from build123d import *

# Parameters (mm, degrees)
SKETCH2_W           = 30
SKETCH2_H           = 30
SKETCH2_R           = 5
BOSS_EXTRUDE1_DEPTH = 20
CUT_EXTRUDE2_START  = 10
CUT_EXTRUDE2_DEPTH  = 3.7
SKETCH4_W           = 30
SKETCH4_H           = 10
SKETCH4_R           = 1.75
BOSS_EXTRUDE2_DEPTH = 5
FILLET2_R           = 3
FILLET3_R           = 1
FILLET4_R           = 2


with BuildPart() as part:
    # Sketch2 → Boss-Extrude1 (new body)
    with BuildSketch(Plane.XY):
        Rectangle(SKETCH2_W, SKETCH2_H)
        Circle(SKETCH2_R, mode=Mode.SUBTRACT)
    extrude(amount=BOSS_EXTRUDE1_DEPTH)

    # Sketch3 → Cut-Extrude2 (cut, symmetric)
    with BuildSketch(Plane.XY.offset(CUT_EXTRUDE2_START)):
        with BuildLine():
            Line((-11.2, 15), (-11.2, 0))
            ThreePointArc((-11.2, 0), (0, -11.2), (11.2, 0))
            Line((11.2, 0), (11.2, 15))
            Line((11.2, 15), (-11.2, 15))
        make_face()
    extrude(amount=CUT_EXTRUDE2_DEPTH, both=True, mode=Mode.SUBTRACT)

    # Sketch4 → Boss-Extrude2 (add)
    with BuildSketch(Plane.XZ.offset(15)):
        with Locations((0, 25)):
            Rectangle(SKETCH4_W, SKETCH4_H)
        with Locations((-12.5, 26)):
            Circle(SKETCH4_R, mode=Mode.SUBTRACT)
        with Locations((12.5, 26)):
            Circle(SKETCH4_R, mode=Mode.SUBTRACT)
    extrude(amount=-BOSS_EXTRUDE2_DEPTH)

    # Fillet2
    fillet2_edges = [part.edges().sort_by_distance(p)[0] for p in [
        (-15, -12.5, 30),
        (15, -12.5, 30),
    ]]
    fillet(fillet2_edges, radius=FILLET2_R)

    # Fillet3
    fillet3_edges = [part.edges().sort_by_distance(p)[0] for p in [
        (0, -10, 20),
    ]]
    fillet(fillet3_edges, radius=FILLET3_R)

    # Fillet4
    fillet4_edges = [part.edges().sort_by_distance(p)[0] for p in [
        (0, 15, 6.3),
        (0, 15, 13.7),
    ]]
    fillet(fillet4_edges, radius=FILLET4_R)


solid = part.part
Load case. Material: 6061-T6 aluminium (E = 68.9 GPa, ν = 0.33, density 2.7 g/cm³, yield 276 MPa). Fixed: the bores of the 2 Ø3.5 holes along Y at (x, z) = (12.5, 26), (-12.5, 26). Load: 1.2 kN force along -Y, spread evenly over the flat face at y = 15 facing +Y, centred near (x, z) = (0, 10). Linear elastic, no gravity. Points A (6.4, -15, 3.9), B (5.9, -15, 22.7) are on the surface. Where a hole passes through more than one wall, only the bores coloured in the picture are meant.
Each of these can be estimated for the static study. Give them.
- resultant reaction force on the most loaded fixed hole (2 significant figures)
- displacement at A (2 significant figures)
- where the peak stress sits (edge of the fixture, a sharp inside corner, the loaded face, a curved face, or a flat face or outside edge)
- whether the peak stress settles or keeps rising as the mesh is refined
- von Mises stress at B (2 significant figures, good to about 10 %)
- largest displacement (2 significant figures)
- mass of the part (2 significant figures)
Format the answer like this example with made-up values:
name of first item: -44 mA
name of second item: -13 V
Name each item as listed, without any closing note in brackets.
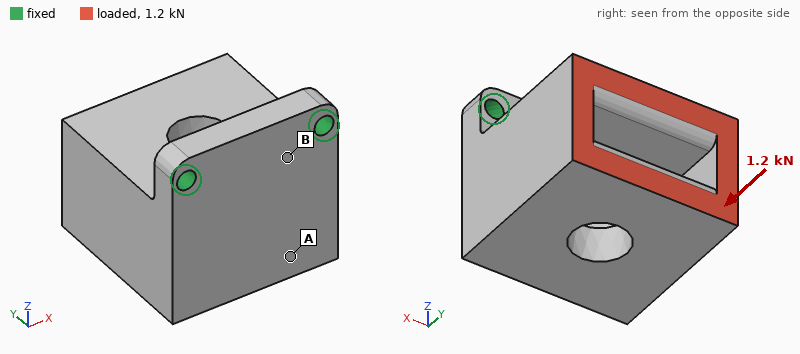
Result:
resultant reaction force on the most loaded fixed hole: 600 N
displacement at A: 0.13 mm
where the peak stress sits: edge of the fixture
whether the peak stress settles or keeps rising as the mesh is refined: keeps rising
von Mises stress at B: 73 MPa
largest displacement: 0.24 mm
mass of the part: 39 g
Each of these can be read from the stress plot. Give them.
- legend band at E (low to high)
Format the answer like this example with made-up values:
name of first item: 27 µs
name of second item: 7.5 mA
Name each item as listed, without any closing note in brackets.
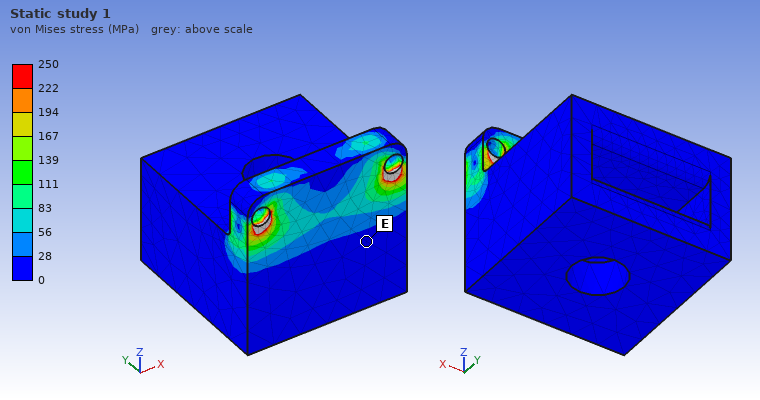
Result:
legend band at E: 0 to 28 MPa
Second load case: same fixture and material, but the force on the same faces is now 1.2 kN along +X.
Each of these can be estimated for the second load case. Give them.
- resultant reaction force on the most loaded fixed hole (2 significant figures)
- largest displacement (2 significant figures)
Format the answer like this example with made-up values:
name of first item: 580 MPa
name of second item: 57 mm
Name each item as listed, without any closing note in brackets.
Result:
resultant reaction force on the most loaded fixed hole: 1.6 kN
largest displacement: 73 µm
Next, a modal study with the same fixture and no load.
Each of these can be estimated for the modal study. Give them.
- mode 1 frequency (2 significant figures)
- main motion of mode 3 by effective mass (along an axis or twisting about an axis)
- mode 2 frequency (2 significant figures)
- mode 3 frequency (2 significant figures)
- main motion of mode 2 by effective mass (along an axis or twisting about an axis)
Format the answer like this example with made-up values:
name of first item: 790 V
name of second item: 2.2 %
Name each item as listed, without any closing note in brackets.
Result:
mode 1 frequency: 2000 Hz
main motion of mode 3 by effective mass: along X
mode 2 frequency: 5900 Hz
mode 3 frequency: 12 kHz
main motion of mode 2 by effective mass: along X
